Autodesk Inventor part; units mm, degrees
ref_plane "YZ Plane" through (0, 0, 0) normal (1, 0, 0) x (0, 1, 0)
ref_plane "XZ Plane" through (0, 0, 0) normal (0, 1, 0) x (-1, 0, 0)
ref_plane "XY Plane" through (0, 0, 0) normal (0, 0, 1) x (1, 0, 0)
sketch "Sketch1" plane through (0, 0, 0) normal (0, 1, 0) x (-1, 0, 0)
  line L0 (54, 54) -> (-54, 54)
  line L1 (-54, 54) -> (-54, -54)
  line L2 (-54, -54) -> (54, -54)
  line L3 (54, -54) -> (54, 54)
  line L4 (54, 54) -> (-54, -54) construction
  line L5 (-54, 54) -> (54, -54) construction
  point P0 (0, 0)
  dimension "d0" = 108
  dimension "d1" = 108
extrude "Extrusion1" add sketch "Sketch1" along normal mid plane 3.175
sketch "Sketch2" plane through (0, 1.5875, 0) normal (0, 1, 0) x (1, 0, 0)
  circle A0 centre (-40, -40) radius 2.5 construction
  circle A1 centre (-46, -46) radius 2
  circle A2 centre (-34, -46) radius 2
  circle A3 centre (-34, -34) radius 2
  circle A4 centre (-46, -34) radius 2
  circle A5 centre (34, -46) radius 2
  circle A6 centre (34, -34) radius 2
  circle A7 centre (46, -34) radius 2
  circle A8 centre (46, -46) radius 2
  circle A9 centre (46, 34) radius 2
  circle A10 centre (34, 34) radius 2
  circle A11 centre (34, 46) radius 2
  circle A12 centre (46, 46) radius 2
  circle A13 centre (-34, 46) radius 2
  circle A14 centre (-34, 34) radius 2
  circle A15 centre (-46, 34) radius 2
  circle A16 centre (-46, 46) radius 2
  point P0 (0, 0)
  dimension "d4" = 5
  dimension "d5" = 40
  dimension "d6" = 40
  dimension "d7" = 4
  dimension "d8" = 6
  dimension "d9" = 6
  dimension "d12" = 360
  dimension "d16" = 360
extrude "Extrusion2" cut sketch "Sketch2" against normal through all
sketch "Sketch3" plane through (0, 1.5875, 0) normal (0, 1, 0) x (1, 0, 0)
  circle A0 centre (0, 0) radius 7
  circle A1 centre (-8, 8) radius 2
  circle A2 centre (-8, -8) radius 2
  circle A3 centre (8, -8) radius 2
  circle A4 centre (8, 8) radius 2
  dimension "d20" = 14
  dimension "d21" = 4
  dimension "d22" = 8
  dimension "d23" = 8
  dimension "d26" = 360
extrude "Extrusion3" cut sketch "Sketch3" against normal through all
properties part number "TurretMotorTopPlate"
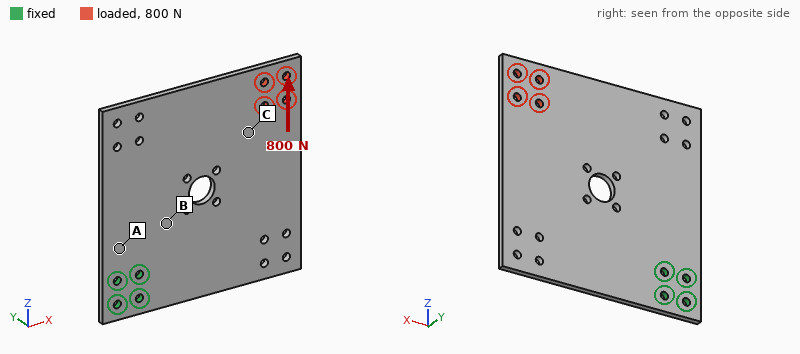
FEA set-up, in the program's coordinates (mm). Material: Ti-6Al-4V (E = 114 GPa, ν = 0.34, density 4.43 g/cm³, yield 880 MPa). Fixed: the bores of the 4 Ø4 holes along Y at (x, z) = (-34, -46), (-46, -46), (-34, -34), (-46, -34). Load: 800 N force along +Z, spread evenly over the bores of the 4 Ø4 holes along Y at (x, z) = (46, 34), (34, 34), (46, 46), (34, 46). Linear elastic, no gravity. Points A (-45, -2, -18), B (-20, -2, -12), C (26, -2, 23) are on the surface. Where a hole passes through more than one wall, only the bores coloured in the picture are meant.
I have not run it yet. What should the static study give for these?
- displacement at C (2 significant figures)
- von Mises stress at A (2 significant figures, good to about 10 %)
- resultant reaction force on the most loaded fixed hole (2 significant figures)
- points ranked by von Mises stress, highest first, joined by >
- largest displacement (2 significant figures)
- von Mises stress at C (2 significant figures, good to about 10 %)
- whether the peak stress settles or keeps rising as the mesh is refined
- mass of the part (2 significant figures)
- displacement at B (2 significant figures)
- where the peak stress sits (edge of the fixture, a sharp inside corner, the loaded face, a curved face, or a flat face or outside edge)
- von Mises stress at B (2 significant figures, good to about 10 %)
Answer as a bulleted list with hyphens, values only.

- 0.076 mm
- 24 MPa
- 2.2 kN
- A > B > C
- 0.12 mm
- 6.8 MPa
- keeps rising
- 160 g
- 0.025 mm
- edge of the fixture
- 14 MPa
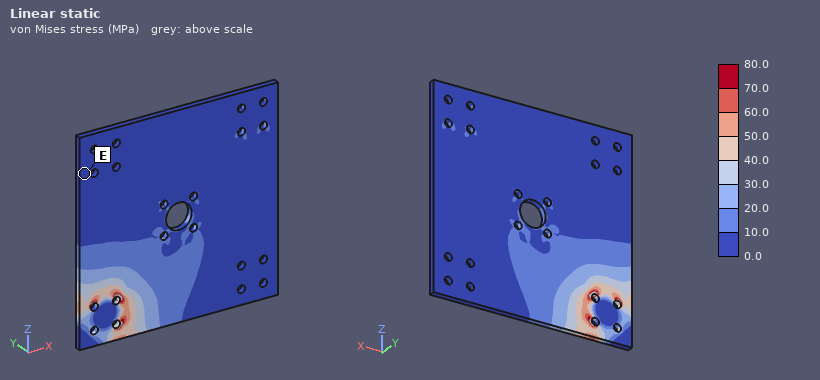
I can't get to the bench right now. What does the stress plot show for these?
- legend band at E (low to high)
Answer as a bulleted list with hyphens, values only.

- 0.0 to 10.0 MPa
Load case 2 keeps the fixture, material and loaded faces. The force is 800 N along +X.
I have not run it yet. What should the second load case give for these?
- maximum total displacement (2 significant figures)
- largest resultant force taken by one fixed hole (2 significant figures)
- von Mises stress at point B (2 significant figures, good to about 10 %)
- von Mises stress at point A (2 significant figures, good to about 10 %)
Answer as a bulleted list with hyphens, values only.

- 0.12 mm
- 2.2 kN
- 13 MPa
- 29 MPa
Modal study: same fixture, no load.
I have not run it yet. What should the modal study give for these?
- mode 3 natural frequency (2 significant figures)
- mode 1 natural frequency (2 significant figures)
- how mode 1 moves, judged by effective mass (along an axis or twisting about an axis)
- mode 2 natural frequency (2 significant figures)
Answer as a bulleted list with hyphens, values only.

- 790 Hz
- 200 Hz
- along Y
- 360 Hz
